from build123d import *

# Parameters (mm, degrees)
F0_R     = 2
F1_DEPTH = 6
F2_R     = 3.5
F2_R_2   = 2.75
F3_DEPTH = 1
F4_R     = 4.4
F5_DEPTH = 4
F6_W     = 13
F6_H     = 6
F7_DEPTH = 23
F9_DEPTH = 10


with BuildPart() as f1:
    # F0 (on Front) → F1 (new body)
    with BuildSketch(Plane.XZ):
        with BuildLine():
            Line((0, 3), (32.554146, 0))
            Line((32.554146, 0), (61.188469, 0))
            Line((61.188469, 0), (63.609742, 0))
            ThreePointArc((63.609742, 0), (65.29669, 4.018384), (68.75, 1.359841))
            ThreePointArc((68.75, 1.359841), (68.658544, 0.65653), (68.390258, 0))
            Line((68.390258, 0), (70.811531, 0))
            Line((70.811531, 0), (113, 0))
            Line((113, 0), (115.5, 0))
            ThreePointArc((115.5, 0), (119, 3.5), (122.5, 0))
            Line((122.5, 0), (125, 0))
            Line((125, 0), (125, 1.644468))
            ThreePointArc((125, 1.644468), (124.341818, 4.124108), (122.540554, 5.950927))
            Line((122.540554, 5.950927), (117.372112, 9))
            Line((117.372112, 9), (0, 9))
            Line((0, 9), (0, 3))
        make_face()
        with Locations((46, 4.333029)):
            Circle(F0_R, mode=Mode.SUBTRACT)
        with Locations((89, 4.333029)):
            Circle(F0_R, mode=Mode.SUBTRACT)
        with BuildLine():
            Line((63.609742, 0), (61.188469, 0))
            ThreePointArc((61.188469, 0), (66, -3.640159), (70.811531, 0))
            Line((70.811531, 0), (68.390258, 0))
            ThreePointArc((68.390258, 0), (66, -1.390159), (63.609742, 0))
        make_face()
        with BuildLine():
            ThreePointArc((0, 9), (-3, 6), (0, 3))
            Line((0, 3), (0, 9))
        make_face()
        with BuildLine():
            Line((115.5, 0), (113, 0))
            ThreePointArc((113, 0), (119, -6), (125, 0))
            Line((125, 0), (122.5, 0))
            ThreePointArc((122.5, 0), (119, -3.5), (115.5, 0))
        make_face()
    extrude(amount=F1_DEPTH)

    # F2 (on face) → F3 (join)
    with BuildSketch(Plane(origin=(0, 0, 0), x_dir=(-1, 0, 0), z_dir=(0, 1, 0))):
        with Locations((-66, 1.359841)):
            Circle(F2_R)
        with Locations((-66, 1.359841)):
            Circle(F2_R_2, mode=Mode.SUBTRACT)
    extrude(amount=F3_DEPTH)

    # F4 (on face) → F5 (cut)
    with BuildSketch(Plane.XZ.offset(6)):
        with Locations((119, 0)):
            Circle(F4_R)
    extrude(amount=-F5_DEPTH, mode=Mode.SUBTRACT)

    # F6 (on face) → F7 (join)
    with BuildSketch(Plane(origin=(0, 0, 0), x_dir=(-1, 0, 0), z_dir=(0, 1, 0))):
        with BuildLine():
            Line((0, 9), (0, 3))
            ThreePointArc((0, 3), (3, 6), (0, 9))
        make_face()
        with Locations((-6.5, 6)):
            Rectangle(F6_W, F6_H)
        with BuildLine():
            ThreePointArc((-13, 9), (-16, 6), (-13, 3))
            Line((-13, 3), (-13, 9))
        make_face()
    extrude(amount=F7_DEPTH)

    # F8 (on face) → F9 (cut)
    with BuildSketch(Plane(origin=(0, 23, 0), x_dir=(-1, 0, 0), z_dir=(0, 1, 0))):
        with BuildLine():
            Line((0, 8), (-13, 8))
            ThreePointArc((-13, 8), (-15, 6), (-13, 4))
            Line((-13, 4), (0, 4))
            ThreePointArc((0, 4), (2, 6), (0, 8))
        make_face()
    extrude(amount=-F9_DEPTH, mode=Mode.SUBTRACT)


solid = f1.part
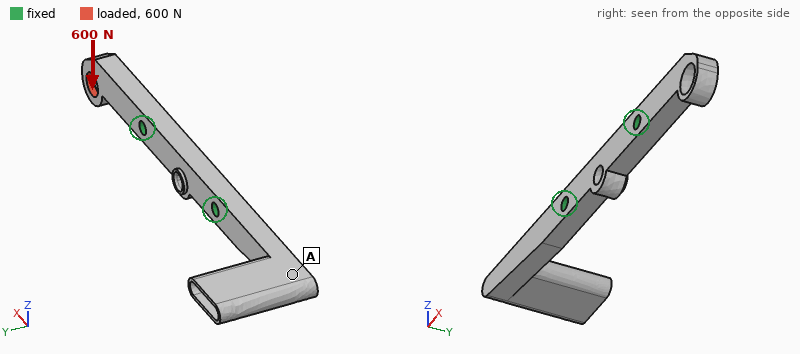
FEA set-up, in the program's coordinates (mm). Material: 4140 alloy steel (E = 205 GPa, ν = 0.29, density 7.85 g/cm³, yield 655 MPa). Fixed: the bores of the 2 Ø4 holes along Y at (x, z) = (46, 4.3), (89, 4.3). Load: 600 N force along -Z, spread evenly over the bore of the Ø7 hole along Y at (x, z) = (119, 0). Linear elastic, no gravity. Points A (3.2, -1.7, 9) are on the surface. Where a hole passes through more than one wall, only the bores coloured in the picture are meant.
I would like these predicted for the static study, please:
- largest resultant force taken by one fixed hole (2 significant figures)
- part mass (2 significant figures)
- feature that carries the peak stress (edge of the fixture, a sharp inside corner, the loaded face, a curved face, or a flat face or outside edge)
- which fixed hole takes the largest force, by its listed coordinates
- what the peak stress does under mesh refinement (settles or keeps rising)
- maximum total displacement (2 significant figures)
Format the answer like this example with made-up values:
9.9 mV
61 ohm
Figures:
670 N
64 g
edge of the fixture
(89, 4.3)
keeps rising
0.12 mm
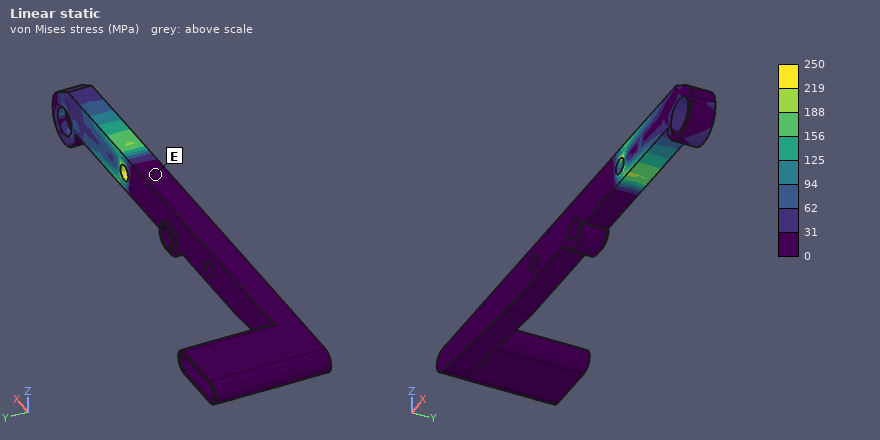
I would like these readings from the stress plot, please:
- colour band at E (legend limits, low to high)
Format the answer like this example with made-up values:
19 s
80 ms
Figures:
0 to 31 MPa
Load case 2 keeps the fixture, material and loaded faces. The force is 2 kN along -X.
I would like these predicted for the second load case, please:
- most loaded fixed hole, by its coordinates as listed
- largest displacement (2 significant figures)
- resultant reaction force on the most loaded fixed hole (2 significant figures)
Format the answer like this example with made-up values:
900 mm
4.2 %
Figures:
(89, 4.3)
0.13 mm
2.0 kN
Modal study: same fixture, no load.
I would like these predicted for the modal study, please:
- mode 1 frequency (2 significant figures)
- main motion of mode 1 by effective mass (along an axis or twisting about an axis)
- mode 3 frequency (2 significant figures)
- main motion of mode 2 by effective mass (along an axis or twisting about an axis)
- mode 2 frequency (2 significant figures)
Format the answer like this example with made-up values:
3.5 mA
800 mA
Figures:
1300 Hz
along Y
4300 Hz
along Z
1700 Hz
